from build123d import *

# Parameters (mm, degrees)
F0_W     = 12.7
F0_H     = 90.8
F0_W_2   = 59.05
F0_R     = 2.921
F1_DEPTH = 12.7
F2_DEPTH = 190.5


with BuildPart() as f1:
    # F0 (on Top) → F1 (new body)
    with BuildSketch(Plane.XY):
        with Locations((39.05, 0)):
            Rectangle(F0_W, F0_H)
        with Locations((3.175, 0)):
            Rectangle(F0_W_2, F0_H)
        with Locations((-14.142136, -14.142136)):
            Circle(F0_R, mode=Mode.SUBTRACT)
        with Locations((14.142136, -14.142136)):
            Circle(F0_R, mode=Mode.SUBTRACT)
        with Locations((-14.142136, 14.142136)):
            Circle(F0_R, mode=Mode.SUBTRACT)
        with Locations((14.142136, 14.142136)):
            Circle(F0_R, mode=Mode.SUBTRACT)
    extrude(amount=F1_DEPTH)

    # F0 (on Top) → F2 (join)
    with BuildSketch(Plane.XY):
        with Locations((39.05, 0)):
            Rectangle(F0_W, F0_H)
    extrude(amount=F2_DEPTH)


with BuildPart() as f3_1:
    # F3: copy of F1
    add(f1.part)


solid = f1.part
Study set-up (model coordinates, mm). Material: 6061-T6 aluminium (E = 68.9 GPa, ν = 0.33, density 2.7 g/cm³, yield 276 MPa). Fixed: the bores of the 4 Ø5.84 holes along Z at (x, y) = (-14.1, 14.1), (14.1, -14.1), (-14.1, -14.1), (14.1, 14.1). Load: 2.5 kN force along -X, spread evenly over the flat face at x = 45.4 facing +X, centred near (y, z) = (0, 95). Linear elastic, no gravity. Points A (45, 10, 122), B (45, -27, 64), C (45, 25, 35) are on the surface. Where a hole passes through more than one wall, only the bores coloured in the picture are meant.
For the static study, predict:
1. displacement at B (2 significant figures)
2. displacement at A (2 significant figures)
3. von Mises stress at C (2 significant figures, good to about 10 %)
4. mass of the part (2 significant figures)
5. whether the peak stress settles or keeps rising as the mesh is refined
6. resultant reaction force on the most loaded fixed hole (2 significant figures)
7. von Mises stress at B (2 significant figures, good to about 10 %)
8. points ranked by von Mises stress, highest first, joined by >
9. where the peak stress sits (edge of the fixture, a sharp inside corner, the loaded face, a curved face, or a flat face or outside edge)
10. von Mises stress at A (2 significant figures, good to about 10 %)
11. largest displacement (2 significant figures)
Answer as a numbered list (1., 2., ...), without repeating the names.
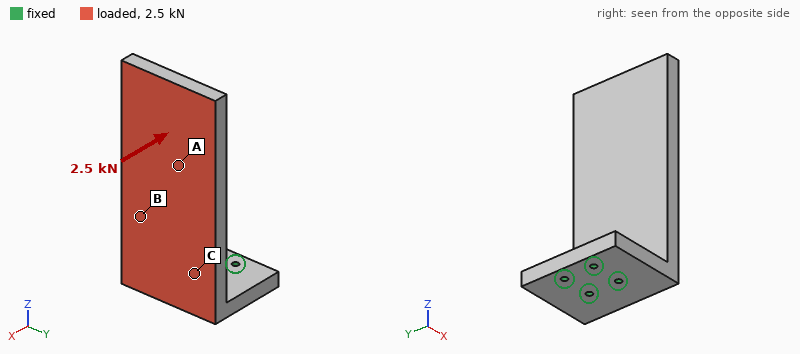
1. 0.56 mm
2. 1.4 mm
3. 61 MPa
4. 770 g
5. keeps rising
6. 2.1 kN
7. 42 MPa
8. C > B > A
9. edge of the fixture
10. 13 MPa
11. 2.6 mm
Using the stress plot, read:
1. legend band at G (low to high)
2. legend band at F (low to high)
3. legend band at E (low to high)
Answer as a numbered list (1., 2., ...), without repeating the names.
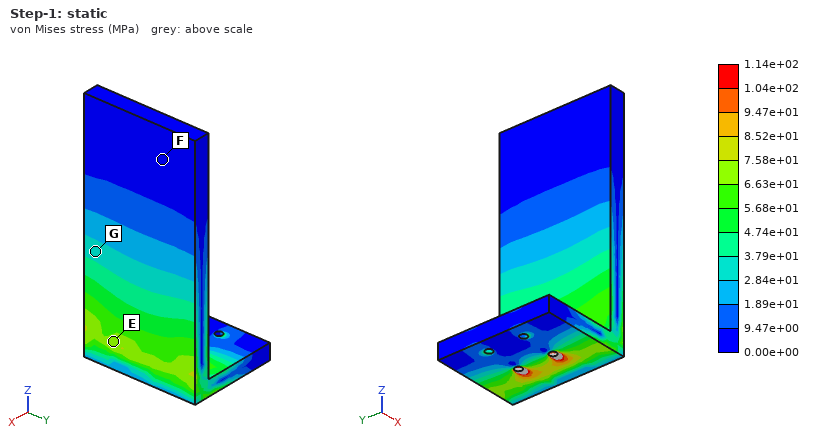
1. 2.84e+01 to 3.79e+01 MPa
2. 0.00e+00 to 9.47e+00 MPa
3. 6.63e+01 to 7.58e+01 MPa
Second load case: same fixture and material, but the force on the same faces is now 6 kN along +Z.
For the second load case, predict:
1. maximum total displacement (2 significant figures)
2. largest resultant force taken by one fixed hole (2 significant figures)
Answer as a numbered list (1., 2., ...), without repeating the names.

1. 0.94 mm
2. 4.2 kN
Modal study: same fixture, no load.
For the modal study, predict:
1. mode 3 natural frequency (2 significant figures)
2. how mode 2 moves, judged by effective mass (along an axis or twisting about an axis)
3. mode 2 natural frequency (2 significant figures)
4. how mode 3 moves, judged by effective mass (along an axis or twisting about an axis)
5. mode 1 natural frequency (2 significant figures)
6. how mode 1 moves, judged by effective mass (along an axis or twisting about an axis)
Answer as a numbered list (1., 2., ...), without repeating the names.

1. 1200 Hz
2. along Y
3. 620 Hz
4. twisting about Z
5. 250 Hz
6. along X
